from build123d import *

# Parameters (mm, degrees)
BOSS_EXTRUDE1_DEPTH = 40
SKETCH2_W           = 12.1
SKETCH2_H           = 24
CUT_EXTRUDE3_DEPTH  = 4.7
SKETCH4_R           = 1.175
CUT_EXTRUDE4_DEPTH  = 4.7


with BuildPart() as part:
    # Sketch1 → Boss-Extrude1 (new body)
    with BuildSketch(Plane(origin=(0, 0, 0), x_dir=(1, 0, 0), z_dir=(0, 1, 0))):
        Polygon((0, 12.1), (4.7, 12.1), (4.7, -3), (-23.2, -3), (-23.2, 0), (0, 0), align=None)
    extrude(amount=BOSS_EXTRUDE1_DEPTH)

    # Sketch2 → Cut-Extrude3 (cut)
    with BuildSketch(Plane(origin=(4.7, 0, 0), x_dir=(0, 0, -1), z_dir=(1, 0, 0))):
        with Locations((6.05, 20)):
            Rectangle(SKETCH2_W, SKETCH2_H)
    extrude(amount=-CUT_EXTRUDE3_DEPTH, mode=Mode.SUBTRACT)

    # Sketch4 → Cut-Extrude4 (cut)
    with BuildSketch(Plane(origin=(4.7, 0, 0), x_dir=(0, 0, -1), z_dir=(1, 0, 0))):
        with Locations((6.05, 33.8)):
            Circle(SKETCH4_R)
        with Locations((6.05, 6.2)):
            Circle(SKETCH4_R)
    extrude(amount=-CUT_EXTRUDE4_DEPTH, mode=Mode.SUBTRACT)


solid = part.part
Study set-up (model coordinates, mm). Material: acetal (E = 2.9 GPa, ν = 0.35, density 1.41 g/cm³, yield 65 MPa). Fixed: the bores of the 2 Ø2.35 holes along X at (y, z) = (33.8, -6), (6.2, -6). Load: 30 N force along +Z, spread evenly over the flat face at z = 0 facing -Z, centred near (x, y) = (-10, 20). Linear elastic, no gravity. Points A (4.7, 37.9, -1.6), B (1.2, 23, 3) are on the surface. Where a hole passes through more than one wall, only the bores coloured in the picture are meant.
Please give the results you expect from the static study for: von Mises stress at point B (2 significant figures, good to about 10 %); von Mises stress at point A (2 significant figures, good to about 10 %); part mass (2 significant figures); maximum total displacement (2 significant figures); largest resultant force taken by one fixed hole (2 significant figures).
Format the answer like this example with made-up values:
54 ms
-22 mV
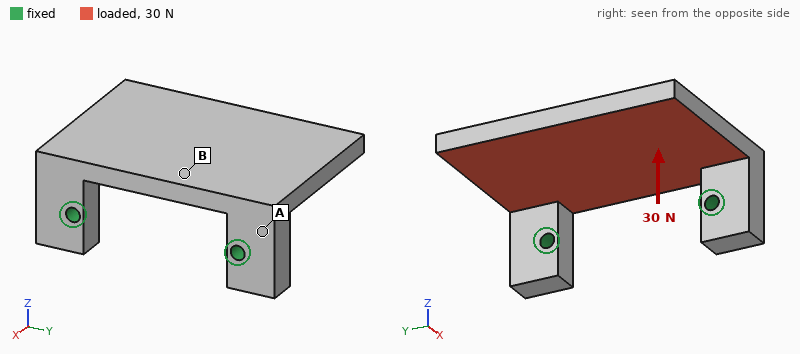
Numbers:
1.5 MPa
4.7 MPa
5.9 g
0.48 mm
16 N
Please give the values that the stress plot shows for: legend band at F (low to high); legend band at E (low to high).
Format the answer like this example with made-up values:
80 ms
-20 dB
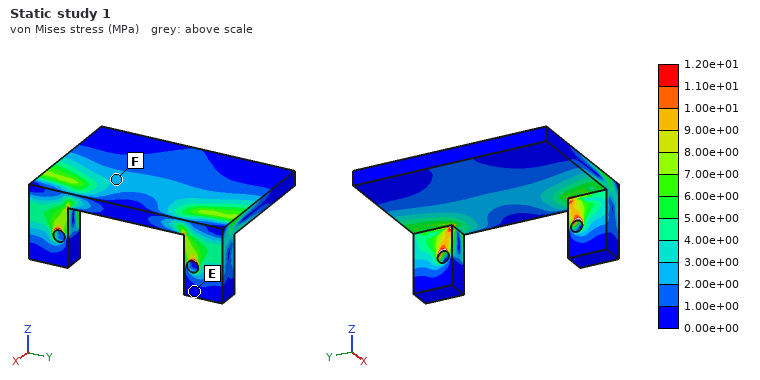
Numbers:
2.00e+00 to 3.00e+00 MPa
0.00e+00 to 1.00e+00 MPa
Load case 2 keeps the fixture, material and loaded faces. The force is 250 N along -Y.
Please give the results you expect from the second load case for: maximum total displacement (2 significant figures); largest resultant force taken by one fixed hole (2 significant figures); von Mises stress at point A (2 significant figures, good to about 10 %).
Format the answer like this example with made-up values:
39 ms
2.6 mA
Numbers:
0.40 mm
160 N
7.2 MPa
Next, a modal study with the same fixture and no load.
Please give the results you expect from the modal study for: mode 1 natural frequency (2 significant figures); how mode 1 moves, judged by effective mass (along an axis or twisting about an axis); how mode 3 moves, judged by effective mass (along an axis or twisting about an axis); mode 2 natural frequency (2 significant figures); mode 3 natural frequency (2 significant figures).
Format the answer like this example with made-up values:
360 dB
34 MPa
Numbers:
750 Hz
along Z
along Y
1700 Hz
2600 Hz
